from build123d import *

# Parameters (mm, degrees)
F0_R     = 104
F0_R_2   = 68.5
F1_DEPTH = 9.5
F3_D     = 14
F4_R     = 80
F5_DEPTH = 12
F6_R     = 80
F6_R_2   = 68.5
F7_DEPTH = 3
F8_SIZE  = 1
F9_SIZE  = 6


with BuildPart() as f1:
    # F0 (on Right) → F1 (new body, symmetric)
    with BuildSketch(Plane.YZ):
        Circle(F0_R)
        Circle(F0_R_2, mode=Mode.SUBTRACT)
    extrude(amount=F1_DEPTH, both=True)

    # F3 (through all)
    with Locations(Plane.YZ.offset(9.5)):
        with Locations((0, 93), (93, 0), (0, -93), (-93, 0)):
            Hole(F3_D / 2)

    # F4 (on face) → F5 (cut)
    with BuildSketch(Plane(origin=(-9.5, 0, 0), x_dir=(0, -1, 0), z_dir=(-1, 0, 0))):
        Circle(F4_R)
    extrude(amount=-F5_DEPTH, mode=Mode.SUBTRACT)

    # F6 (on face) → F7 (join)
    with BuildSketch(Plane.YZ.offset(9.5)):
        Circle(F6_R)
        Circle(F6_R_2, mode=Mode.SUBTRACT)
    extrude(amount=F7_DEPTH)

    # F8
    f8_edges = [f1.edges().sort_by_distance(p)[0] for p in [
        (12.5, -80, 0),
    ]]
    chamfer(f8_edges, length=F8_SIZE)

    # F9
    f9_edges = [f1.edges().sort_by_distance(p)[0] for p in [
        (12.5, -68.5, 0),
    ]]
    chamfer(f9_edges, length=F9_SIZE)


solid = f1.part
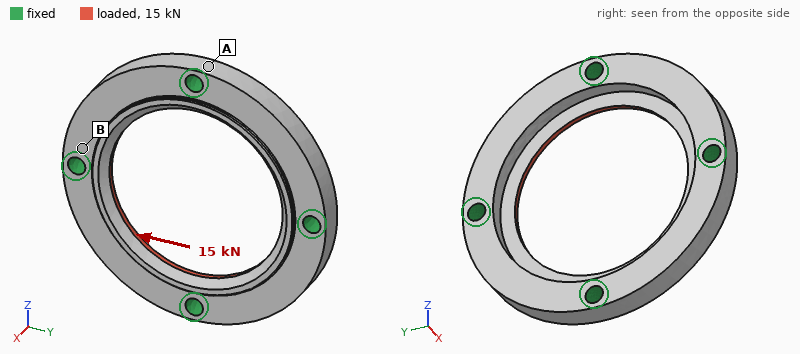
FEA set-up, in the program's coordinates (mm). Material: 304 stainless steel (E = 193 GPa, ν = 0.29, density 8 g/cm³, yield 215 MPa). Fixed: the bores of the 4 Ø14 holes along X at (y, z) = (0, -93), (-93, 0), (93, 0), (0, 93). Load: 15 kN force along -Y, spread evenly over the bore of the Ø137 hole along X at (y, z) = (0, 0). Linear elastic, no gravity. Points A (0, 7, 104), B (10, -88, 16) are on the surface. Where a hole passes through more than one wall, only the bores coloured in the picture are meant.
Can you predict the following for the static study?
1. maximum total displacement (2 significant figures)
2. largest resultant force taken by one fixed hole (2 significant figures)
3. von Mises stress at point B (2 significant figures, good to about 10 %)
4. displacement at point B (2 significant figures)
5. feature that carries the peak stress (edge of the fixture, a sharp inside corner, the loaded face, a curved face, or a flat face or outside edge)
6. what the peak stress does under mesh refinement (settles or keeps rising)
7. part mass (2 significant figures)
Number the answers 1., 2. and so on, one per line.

1. 3.3 µm
2. 4.9 kN
3. 7.8 MPa
4. 0.87 µm
5. edge of the fixture
6. keeps rising
7. 2.4 kg
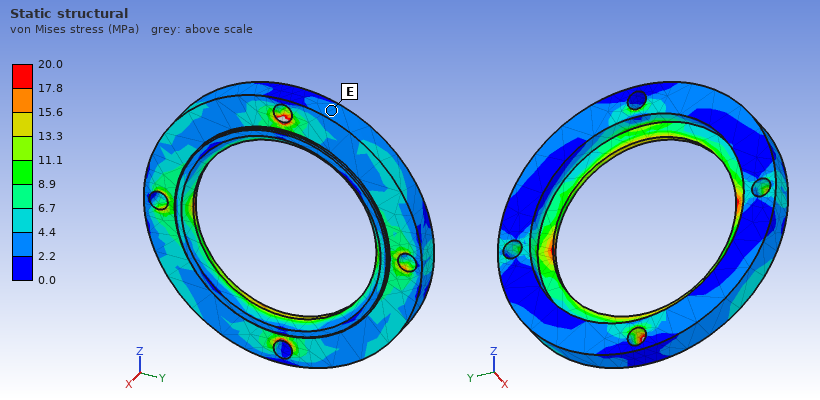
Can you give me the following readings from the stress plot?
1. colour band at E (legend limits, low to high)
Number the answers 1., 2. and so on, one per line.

1. 2.2 to 4.4 MPa
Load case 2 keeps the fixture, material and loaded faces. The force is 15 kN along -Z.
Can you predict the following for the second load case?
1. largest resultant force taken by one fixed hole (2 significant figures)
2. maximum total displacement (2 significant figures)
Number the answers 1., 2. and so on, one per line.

1. 4.9 kN
2. 3.3 µm
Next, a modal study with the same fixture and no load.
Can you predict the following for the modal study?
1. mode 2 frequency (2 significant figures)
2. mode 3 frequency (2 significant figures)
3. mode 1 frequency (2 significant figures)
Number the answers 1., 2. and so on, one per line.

1. 4400 Hz
2. 4400 Hz
3. 4300 Hz
